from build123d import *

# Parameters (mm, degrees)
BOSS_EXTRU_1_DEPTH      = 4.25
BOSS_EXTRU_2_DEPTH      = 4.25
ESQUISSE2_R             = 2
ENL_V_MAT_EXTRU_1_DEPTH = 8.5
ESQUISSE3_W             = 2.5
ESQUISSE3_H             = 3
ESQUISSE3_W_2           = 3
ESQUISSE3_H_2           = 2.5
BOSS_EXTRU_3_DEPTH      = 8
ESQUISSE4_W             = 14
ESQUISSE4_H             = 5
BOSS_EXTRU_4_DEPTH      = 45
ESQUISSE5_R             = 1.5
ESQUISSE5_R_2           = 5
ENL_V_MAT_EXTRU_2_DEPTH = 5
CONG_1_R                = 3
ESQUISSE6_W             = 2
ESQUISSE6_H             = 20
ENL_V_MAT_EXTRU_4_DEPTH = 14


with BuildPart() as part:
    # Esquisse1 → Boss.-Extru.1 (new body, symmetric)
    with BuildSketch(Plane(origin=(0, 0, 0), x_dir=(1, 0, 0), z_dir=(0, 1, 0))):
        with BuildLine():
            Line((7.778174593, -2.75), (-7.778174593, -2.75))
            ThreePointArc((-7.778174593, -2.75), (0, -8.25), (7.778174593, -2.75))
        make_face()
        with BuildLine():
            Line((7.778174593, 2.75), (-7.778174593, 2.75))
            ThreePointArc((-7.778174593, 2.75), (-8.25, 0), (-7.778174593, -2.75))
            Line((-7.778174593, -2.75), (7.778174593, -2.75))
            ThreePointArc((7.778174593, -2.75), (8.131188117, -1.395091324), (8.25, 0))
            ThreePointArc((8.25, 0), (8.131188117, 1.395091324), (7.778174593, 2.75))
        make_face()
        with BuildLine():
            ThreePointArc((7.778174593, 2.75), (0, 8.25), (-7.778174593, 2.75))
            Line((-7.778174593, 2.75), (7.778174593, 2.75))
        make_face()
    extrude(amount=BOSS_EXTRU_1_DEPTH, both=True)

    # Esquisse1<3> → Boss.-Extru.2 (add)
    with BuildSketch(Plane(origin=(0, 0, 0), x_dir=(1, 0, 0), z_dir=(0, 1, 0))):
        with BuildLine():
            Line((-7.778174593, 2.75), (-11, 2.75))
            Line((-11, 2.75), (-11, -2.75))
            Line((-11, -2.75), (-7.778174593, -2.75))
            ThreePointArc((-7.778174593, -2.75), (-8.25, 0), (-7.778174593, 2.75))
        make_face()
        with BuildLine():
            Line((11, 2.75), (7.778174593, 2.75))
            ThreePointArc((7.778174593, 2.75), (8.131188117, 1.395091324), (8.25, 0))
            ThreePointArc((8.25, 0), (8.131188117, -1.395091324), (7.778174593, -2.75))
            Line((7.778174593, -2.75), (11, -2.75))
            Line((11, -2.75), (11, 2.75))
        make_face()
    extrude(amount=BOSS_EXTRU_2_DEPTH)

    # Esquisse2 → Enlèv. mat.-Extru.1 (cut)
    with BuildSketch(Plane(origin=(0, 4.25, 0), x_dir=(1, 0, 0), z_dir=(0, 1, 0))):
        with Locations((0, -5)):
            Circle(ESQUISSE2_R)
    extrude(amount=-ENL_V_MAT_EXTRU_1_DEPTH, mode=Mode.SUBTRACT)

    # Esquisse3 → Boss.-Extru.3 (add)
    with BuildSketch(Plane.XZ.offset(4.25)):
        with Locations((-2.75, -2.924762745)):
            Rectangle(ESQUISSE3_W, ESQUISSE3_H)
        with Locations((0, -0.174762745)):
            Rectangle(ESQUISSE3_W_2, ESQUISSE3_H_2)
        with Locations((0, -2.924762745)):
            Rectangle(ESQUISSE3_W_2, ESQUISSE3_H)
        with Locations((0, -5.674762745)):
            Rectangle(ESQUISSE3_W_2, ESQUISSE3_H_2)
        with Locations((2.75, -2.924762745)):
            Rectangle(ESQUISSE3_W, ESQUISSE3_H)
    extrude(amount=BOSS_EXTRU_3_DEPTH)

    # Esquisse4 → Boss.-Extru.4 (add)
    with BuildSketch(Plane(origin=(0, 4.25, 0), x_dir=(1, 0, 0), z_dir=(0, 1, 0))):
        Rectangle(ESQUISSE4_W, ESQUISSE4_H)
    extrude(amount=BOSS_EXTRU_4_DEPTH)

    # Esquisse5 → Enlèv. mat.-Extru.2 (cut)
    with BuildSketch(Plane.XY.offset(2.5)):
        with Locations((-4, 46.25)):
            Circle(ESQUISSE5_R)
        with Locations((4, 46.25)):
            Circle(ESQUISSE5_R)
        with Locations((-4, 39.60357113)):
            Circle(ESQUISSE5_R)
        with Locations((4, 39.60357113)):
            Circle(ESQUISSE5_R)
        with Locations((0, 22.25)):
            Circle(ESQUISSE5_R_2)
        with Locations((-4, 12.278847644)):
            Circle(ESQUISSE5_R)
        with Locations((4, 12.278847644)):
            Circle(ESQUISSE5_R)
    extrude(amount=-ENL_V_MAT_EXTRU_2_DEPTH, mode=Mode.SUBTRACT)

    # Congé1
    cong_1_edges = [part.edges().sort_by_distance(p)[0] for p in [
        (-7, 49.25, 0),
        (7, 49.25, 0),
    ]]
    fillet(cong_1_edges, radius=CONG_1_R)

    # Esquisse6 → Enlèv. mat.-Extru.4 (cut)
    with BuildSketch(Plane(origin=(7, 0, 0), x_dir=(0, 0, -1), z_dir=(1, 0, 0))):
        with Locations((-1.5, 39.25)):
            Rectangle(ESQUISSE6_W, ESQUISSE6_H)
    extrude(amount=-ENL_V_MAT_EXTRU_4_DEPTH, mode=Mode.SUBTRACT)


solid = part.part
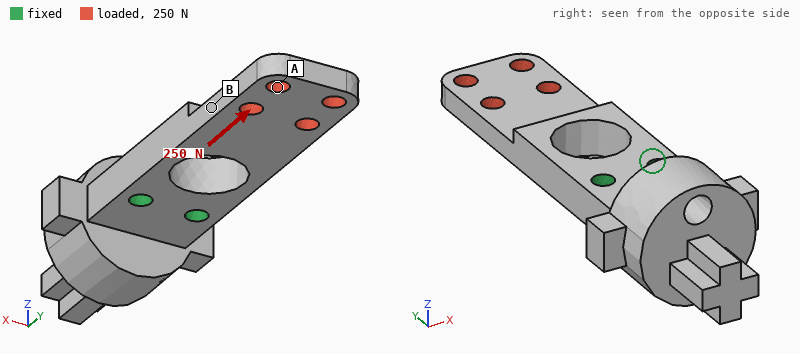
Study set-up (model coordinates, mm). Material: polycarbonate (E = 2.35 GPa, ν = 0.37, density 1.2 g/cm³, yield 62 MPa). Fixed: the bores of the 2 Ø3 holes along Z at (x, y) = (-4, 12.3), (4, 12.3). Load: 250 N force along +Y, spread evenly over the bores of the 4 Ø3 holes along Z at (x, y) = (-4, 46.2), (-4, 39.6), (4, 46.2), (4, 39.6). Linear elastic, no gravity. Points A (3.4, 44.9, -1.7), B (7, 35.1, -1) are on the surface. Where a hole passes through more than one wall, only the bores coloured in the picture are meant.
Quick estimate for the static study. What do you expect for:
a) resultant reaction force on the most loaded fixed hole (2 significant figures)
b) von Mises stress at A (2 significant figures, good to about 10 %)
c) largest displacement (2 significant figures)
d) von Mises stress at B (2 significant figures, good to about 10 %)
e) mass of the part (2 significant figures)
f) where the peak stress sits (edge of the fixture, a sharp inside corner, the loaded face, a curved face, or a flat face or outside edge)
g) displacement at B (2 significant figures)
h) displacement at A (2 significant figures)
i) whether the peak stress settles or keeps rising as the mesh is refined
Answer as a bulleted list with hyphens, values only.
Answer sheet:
- 130 N
- 3.3 MPa
- 0.78 mm
- 8.5 MPa
- 5.0 g
- a sharp inside corner
- 0.39 mm
- 0.66 mm
- keeps rising
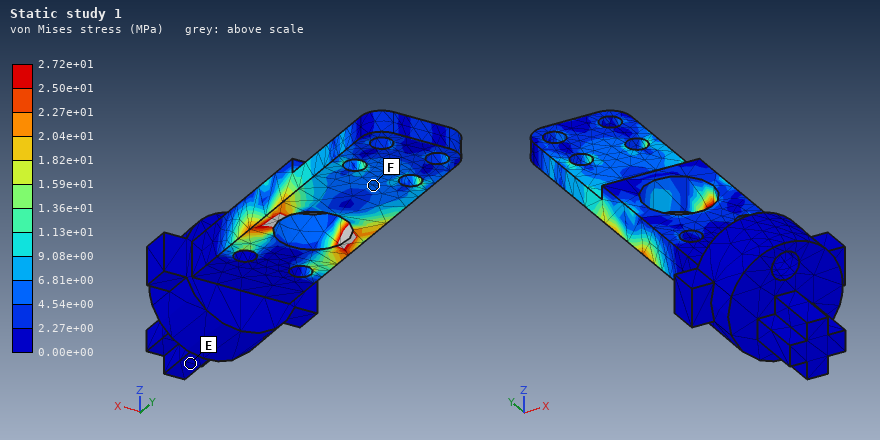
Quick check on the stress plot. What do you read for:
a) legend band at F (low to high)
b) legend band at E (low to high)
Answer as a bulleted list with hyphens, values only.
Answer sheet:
- 4.54e+00 to 6.81e+00 MPa
- 0.00e+00 to 2.27e+00 MPa
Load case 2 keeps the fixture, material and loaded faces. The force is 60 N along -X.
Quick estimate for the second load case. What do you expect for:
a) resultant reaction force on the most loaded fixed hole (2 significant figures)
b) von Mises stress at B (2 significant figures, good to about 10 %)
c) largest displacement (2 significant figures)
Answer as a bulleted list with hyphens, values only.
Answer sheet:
- 180 N
- 5.3 MPa
- 0.59 mm
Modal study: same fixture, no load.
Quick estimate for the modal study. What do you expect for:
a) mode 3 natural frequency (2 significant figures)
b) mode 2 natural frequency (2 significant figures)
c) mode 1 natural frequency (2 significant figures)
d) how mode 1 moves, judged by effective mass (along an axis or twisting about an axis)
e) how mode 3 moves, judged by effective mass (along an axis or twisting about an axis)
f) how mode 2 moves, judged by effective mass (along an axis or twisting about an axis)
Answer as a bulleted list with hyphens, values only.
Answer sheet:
- 2000 Hz
- 1900 Hz
- 760 Hz
- along Z
- along X
- along Z
